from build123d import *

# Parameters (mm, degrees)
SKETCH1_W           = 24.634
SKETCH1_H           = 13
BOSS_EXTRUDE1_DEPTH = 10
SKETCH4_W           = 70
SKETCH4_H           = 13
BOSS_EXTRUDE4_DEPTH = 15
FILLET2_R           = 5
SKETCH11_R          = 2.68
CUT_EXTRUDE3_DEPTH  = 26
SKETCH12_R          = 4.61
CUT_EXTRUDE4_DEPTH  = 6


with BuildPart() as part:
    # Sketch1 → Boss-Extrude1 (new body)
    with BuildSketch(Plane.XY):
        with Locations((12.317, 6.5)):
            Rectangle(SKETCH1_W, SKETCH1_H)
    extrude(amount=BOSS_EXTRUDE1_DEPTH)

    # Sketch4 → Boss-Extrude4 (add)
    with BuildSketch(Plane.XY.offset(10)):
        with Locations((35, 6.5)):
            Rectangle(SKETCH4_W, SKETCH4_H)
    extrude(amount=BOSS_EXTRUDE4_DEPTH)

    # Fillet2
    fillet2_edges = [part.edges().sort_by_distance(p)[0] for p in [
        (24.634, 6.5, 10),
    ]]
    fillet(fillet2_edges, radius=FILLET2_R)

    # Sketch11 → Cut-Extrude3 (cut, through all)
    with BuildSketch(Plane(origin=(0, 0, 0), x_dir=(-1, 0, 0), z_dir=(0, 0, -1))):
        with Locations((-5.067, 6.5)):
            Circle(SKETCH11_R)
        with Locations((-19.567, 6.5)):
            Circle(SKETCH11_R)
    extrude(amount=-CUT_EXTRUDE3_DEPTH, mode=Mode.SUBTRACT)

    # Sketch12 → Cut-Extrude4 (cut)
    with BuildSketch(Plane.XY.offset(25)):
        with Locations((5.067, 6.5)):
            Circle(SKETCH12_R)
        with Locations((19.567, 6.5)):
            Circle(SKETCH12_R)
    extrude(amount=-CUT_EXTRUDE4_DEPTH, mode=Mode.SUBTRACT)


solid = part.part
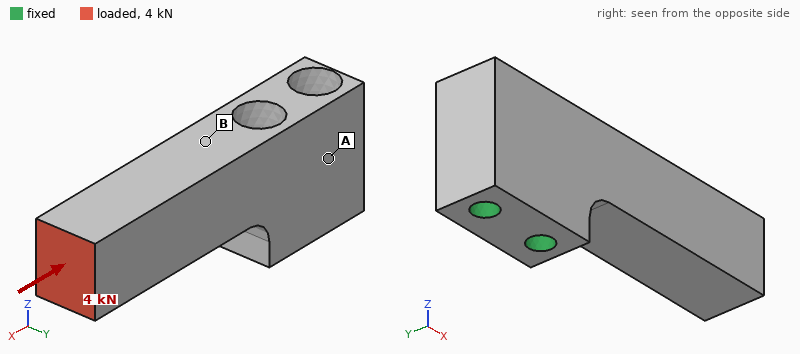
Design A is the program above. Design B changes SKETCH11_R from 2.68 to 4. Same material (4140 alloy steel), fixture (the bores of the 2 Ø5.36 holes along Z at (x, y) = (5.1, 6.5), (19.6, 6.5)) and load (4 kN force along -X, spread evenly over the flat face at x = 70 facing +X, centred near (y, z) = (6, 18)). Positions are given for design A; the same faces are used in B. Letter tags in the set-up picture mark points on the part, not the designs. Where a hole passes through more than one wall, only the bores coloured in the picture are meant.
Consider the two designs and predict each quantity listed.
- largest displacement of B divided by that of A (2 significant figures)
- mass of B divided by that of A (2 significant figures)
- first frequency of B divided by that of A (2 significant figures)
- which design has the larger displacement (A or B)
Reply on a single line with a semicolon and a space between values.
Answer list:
0.86; 0.93; 1.1; A
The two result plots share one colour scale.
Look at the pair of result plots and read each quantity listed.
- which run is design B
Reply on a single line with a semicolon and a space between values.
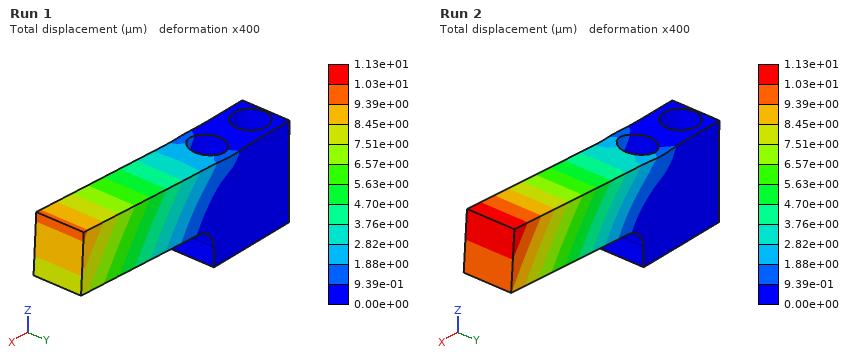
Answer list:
Run 1
